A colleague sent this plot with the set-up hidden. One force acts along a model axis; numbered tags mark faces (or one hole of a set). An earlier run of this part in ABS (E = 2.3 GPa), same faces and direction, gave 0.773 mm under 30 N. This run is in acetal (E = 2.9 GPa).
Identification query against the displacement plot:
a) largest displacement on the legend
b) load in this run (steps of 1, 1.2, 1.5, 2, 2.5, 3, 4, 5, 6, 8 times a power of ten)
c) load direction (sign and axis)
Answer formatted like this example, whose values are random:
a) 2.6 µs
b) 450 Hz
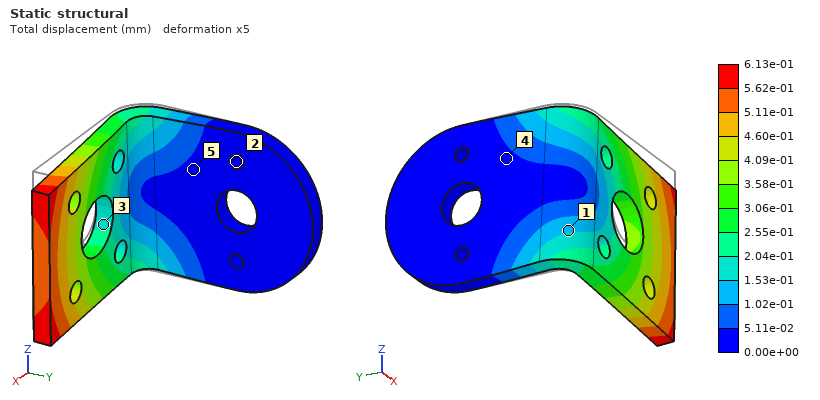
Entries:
a) 6.13e-01 mm
b) 30 N
c) -Z
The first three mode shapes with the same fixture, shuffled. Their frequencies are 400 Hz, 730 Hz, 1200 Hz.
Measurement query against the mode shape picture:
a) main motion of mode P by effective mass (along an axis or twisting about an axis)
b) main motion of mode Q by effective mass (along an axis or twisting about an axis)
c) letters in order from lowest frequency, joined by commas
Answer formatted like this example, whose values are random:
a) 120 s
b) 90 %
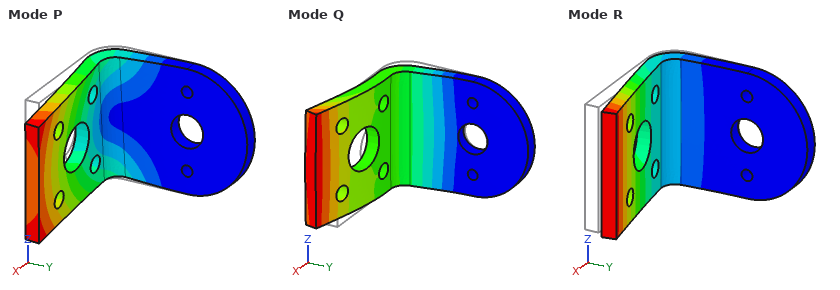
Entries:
a) along Z
b) along X
c) R, P, Q
